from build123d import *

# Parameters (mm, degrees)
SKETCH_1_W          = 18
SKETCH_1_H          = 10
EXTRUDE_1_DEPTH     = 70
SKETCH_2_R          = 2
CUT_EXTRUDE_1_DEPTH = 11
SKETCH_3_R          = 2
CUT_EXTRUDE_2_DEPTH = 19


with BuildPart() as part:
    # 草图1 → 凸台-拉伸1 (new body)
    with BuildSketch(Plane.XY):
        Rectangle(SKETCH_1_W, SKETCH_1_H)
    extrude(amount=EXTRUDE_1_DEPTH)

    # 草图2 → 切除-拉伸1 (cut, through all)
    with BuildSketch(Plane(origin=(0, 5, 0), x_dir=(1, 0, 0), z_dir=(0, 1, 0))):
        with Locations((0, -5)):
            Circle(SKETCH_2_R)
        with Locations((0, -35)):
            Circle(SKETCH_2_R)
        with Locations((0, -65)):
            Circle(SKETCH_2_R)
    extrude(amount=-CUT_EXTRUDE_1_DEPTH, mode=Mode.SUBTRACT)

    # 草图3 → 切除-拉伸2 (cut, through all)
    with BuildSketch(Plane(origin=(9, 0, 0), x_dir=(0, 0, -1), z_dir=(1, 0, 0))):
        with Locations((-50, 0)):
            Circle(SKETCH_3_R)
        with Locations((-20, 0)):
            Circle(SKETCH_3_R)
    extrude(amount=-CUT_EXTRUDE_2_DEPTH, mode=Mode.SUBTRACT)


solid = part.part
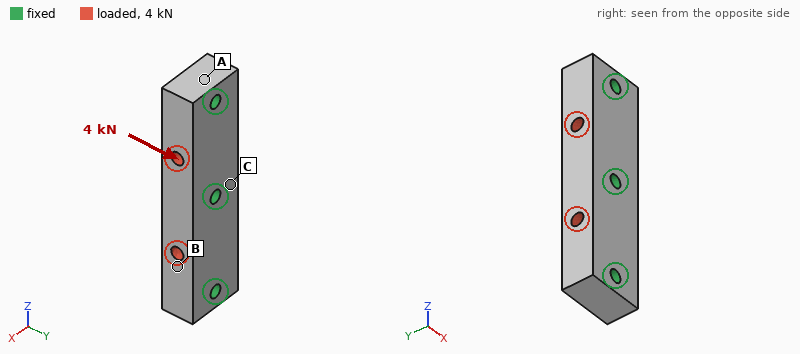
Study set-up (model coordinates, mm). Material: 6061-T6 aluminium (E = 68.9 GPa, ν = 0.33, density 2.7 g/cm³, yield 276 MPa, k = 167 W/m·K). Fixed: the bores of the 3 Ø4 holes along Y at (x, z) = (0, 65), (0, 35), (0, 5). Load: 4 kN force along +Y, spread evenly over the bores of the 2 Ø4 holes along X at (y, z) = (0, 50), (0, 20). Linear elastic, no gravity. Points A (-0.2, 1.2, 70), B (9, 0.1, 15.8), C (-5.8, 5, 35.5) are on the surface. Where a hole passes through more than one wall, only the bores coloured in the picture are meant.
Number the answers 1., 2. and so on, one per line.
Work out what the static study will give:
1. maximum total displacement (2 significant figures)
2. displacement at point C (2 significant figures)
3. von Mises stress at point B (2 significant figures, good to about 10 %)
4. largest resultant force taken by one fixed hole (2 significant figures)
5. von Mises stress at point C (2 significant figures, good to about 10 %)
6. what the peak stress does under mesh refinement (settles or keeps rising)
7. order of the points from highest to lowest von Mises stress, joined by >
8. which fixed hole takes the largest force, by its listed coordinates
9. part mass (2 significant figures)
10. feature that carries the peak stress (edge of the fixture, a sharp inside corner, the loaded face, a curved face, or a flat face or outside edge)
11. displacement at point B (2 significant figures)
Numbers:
1. 7.0 µm
2. 1.5 µm
3. 13 MPa
4. 2.1 kN
5. 19 MPa
6. keeps rising
7. C > B > A
8. (0, 35)
9. 32 g
10. edge of the fixture
11. 5.6 µm
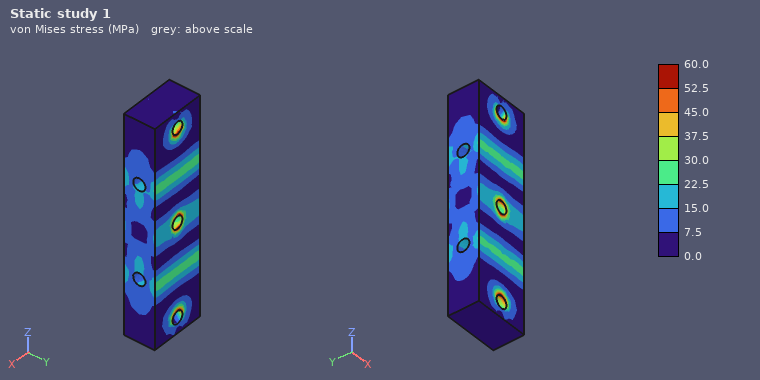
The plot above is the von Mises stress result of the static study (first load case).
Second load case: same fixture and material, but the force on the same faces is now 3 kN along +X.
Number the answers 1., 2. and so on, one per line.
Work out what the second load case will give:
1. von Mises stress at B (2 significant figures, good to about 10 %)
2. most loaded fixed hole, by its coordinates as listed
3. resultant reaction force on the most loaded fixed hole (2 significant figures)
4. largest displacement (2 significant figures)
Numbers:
1. 3.9 MPa
2. (0, 35)
3. 1.8 kN
4. 4.4 µm
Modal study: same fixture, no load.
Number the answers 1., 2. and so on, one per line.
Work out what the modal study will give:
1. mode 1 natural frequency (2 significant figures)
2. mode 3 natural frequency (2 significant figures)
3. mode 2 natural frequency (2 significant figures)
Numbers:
1. 35 kHz
2. 36 kHz
3. 36 kHz
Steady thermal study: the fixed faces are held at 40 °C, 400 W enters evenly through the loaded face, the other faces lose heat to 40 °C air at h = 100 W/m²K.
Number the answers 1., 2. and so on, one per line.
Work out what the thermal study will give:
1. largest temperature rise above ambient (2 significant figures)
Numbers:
1. 53 K
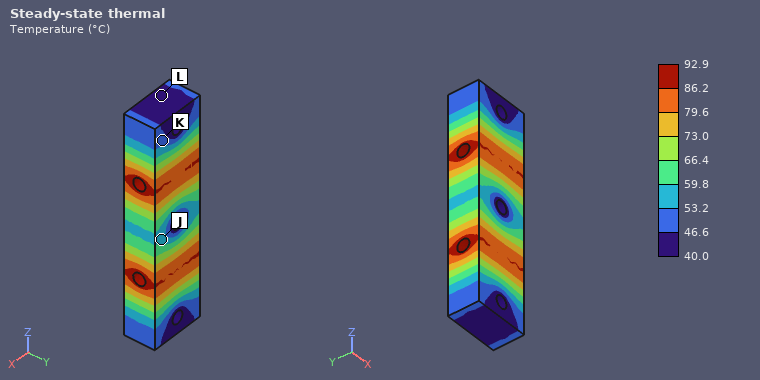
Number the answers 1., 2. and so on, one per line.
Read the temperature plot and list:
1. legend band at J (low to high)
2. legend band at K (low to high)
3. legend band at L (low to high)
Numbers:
1. 53.2 to 59.8 °C
2. 46.6 to 53.2 °C
3. 40.0 to 46.6 °C
